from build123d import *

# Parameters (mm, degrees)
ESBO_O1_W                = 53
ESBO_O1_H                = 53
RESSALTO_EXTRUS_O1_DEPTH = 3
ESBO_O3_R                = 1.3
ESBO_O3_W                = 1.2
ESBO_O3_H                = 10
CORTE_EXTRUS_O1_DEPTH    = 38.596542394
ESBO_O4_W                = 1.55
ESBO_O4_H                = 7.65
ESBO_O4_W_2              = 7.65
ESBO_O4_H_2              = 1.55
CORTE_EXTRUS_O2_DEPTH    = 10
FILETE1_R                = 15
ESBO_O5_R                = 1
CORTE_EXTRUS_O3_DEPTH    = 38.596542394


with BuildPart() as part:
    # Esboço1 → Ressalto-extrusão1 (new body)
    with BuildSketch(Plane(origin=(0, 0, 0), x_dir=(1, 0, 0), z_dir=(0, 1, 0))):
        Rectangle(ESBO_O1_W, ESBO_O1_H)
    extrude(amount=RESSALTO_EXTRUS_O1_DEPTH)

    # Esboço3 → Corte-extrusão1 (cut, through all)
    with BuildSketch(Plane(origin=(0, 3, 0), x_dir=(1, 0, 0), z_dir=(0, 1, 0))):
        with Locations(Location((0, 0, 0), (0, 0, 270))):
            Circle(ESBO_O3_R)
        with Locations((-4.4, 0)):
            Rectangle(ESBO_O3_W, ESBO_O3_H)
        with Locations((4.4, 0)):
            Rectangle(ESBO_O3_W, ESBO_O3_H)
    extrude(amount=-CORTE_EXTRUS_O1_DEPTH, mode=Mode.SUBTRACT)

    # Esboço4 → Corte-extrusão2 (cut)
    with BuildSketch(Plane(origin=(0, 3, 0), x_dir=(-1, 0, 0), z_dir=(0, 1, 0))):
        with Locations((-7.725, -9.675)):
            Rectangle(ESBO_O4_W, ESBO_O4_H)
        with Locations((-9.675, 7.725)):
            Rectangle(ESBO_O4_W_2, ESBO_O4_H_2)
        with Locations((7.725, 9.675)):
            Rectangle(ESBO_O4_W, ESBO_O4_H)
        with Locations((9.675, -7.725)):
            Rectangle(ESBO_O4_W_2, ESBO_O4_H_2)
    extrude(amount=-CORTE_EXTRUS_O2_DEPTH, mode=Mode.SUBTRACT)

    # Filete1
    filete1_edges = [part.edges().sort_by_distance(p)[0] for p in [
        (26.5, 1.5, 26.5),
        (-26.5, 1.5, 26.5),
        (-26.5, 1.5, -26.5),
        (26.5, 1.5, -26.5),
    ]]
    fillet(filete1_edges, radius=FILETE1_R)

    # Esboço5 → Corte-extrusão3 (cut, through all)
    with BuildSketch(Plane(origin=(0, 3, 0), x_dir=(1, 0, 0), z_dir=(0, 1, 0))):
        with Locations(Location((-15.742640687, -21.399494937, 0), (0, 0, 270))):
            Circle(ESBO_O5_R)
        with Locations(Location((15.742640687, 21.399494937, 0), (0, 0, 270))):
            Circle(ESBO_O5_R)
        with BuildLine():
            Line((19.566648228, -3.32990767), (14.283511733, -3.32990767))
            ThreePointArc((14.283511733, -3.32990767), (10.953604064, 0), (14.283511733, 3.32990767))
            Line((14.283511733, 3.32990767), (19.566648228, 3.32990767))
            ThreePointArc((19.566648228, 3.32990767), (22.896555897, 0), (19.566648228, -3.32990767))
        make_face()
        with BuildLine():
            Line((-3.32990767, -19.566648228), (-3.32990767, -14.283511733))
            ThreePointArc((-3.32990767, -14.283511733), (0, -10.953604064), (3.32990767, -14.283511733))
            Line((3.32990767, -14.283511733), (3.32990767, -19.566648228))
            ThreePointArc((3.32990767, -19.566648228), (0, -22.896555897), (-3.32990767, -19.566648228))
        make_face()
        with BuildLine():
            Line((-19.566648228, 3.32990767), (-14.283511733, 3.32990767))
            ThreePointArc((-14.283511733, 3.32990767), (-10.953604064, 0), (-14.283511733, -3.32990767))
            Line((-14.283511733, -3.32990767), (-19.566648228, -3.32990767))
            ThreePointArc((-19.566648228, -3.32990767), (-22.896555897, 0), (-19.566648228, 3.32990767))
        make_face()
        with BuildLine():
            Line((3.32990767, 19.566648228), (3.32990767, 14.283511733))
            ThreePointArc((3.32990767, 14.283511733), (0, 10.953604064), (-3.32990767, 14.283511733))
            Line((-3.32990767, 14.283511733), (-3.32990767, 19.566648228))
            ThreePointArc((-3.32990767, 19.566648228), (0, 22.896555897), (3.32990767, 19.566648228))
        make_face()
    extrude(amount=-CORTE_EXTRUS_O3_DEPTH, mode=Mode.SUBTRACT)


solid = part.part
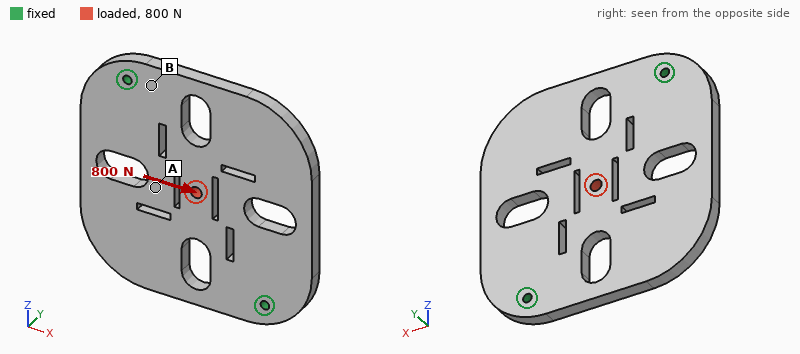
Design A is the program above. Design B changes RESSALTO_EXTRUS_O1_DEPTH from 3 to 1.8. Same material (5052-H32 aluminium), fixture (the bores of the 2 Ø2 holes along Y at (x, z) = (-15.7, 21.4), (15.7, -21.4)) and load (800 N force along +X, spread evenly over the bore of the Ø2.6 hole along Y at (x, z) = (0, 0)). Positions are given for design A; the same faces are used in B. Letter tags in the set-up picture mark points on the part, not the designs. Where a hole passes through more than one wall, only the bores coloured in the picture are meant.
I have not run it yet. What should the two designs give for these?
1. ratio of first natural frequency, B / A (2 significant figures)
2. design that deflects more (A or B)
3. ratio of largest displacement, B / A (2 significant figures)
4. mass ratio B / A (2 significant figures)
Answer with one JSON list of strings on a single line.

["0.63", "B", "1.7", "0.60"]
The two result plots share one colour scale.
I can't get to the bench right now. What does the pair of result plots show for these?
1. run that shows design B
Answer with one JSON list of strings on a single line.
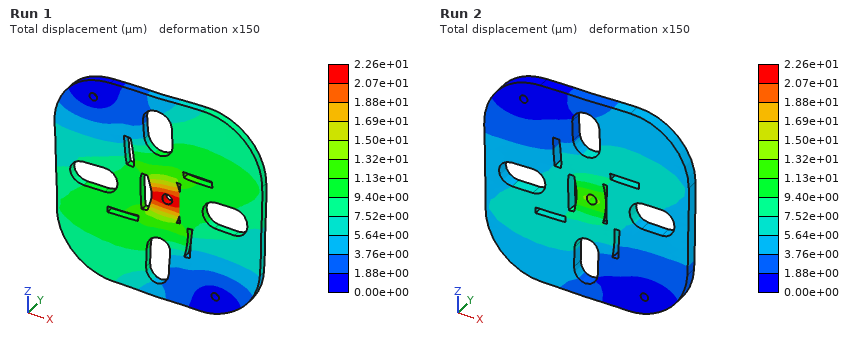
["Run 1"]
